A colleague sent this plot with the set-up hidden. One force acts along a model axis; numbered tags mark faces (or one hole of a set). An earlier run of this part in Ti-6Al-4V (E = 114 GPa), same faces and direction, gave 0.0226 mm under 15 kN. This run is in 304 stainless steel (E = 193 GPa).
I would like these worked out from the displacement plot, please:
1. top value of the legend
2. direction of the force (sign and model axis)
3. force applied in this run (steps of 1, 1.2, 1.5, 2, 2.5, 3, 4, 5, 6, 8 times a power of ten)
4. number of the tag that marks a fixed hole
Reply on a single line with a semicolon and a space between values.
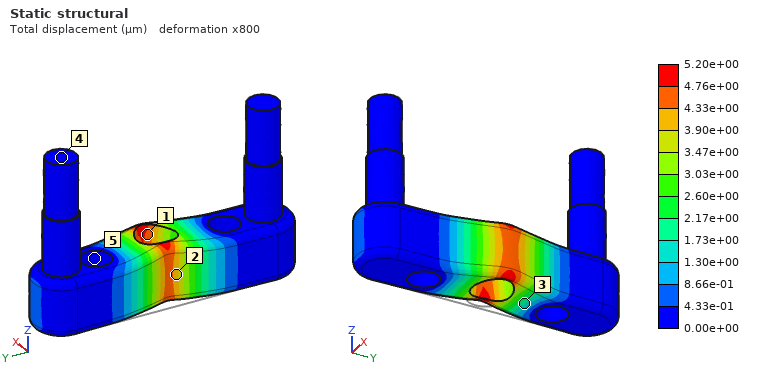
5.20e+00 µm; +X; 6 kN; 5
